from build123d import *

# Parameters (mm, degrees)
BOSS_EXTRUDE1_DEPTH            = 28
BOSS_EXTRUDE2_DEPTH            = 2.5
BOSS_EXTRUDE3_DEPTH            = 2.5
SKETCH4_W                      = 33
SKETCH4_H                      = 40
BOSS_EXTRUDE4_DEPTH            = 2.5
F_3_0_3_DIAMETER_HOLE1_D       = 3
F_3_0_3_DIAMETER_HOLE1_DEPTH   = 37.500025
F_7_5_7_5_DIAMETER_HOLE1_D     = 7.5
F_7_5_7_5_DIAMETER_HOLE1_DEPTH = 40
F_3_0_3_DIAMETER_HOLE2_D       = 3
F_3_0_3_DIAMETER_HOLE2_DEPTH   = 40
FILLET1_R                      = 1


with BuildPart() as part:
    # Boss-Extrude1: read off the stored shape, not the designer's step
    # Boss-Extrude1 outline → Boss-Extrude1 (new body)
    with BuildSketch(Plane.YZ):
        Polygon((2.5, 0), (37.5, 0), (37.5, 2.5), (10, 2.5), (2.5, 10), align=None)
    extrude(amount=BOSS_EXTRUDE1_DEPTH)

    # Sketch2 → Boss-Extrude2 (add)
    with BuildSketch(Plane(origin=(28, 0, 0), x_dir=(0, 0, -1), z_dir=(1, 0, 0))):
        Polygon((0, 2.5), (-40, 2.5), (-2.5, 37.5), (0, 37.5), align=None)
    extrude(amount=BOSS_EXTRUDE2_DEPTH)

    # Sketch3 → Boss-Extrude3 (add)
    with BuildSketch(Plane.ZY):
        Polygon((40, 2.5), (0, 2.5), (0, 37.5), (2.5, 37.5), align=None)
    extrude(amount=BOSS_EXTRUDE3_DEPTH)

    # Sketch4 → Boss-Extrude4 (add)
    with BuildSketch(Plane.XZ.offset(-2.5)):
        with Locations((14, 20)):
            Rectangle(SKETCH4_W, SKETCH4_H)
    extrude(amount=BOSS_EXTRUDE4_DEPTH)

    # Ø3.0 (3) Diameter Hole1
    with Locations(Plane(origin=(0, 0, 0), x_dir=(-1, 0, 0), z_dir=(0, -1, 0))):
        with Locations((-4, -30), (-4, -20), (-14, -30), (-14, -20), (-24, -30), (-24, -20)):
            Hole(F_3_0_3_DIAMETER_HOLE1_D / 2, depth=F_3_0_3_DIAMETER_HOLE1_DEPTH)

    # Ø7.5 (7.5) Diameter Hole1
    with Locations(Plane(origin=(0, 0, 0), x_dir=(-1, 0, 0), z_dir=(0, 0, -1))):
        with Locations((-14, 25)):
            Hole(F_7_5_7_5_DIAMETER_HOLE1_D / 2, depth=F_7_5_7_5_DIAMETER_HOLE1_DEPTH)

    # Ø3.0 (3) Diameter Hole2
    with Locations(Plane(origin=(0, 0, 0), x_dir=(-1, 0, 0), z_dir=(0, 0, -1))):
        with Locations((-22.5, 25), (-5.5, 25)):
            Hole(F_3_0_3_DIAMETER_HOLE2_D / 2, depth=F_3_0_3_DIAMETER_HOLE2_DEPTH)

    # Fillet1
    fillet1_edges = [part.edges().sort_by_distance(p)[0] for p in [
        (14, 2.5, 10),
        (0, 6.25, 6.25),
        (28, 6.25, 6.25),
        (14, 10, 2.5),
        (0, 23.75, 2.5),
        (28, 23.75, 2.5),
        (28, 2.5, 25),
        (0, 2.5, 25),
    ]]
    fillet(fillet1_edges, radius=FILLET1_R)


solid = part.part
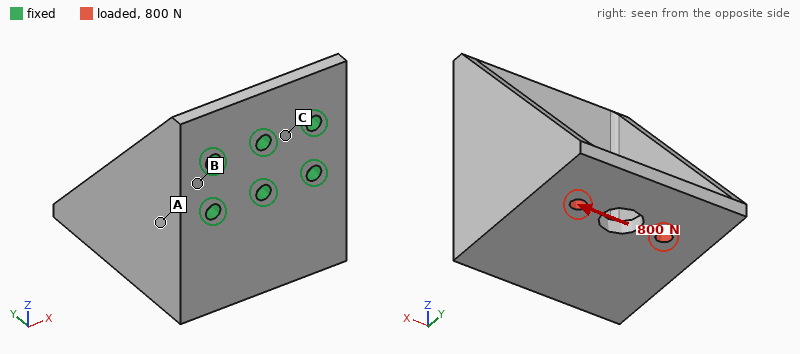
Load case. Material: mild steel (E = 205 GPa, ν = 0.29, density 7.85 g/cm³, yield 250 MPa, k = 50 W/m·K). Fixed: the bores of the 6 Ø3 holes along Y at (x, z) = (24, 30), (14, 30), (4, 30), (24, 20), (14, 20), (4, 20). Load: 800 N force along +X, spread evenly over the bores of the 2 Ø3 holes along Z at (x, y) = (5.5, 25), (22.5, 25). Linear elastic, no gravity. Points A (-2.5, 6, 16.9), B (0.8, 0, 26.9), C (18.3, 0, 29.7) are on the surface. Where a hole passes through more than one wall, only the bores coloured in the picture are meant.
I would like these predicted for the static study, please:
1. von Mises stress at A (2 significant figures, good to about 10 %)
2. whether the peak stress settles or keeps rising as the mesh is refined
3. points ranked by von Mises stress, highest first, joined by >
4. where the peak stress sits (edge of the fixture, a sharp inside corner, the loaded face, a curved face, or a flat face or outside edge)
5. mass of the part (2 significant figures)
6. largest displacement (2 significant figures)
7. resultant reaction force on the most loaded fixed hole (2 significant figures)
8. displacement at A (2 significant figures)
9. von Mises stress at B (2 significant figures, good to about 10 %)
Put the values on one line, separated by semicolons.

41 MPa; keeps rising; B > A > C; edge of the fixture; 79 g; 88 µm; 1.2 kN; 17 µm; 69 MPa
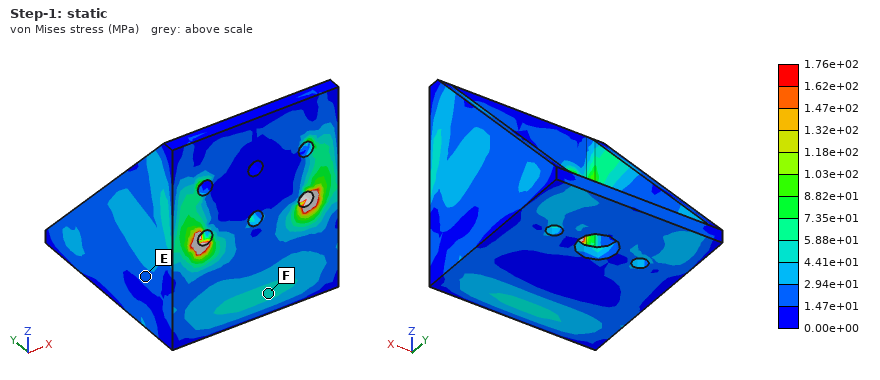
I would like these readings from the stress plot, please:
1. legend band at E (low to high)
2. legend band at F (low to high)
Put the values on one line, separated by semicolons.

1.47e+01 to 2.94e+01 MPa; 4.41e+01 to 5.88e+01 MPa
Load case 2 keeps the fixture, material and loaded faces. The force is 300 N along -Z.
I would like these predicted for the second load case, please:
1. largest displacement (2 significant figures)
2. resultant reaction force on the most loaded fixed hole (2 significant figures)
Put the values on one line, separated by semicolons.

26 µm; 290 N
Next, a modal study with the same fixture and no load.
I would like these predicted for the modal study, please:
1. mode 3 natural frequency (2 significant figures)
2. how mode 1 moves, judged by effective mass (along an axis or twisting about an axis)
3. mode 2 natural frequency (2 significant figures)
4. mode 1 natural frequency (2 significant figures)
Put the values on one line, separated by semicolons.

7500 Hz; along X; 3500 Hz; 3200 Hz
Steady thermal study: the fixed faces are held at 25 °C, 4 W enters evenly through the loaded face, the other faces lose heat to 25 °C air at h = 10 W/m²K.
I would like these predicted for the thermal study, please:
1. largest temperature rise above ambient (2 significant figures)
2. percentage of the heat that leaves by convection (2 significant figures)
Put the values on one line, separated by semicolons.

20 K; 14 %
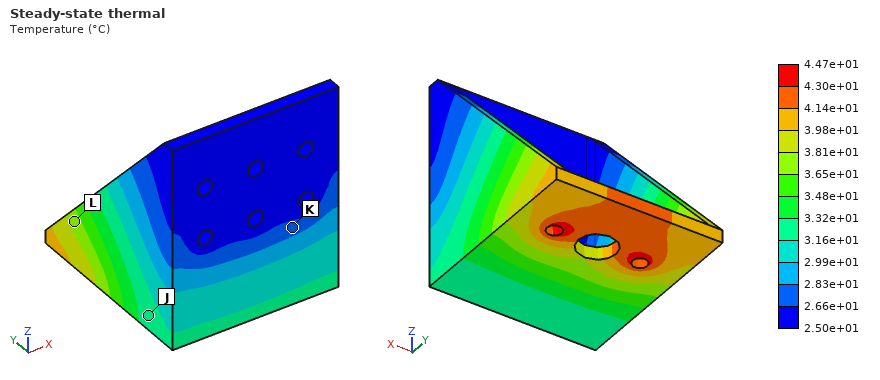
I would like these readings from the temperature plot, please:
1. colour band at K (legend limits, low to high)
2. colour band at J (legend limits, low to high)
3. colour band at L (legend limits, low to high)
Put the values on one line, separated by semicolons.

2.66e+01 to 2.83e+01 °C; 3.16e+01 to 3.32e+01 °C; 3.65e+01 to 3.81e+01 °C
